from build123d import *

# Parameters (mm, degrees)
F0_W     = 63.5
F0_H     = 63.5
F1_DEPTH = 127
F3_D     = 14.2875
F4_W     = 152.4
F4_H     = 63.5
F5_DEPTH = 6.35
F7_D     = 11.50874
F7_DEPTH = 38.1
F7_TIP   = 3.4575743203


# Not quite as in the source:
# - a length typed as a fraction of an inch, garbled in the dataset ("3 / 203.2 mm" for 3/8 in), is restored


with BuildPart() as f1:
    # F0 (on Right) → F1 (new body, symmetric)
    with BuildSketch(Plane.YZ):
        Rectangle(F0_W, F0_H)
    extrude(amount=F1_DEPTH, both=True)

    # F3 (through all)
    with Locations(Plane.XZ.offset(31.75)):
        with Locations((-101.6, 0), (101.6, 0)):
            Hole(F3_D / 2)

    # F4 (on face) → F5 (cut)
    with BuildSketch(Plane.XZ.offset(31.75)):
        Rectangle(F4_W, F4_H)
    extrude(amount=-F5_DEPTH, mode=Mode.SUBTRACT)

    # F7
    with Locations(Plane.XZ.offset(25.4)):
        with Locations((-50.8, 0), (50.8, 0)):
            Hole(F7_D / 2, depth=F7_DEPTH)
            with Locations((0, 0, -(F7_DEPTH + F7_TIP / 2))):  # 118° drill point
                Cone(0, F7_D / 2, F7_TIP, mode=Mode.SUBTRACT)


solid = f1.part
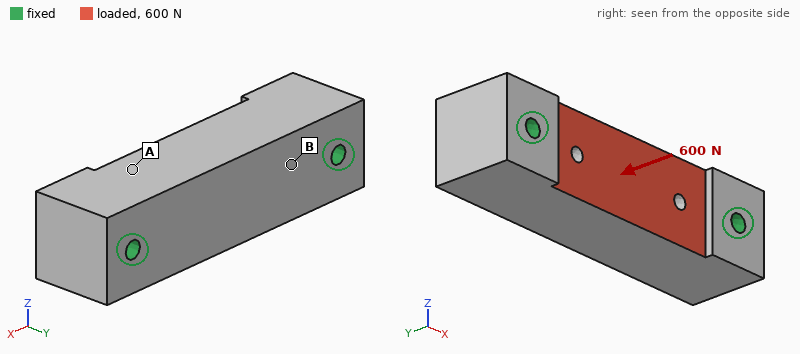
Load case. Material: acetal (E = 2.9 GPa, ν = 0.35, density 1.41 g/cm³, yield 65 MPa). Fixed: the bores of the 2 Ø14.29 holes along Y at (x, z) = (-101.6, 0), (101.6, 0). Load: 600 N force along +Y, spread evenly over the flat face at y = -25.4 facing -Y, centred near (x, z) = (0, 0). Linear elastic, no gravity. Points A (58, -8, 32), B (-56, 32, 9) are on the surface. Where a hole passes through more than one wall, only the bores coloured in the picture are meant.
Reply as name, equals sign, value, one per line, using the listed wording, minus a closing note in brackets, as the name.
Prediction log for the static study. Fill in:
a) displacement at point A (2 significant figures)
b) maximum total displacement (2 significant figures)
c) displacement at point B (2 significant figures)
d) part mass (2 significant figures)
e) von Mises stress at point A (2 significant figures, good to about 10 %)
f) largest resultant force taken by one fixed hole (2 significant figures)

displacement at point A = 6.4 µm
maximum total displacement = 12 µm
displacement at point B = 7.1 µm
part mass = 1.3 kg
von Mises stress at point A = 0.17 MPa
largest resultant force taken by one fixed hole = 300 N
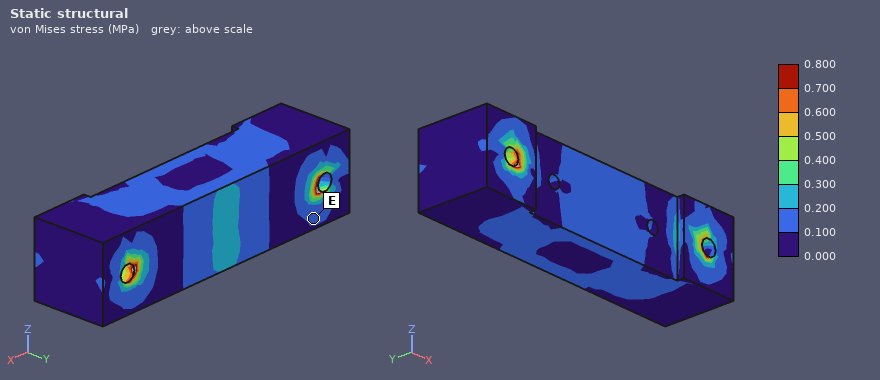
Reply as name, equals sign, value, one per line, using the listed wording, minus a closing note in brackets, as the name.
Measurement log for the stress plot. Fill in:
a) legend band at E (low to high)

legend band at E = 0.100 to 0.200 MPa
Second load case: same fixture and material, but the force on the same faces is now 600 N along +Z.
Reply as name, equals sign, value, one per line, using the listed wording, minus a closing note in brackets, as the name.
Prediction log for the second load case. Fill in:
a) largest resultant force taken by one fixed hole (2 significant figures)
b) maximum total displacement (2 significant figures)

largest resultant force taken by one fixed hole = 300 N
maximum total displacement = 28 µm
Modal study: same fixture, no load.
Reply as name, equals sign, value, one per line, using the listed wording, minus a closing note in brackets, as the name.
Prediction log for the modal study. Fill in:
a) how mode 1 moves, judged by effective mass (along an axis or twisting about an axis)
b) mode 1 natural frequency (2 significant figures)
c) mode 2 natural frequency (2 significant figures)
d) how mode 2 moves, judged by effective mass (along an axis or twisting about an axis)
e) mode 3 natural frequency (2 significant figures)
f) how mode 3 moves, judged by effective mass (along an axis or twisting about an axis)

how mode 1 moves, judged by effective mass = along Z
mode 1 natural frequency = 1100 Hz
mode 2 natural frequency = 1400 Hz
how mode 2 moves, judged by effective mass = along Y
mode 3 natural frequency = 2000 Hz
how mode 3 moves, judged by effective mass = twisting about X
